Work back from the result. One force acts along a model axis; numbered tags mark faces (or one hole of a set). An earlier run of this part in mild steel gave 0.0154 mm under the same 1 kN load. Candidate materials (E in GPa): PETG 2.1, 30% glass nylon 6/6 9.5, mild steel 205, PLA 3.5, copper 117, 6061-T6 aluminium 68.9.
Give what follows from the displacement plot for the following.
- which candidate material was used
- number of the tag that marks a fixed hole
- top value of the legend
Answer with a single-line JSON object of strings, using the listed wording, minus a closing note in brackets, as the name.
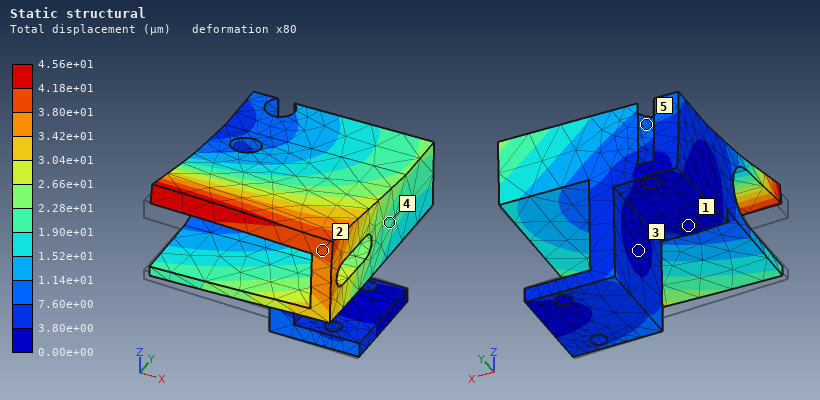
{"which candidate material was used": "6061-T6 aluminium", "number of the tag that marks a fixed hole": "1", "top value of the legend": "4.56e+01 µm"}
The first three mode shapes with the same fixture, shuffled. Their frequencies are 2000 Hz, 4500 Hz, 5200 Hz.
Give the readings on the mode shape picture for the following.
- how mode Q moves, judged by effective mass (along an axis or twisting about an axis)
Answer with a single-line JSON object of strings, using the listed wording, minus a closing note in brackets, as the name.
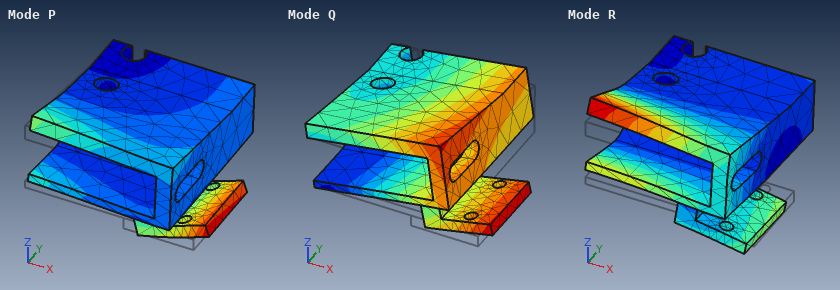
{"how mode Q moves, judged by effective mass": "along Z"}
